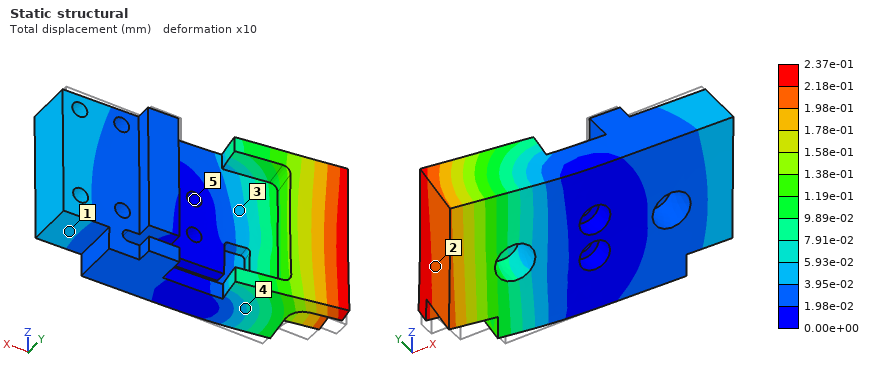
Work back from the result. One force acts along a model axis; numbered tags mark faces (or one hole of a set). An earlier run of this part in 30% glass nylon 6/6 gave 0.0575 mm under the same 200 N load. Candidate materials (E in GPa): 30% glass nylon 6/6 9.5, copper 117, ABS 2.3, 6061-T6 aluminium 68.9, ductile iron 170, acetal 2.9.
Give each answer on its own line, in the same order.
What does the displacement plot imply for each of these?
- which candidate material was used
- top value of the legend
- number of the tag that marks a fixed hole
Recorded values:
ABS
2.37e-01 mm
5
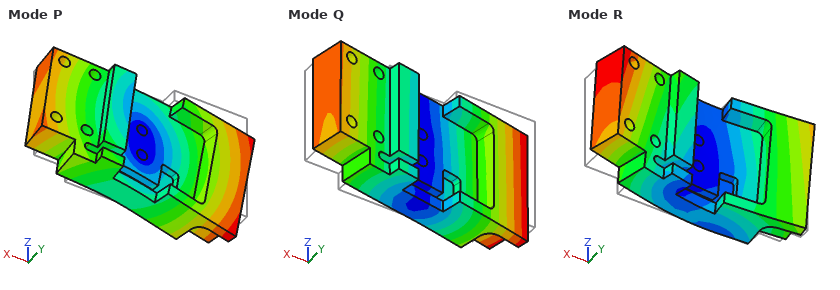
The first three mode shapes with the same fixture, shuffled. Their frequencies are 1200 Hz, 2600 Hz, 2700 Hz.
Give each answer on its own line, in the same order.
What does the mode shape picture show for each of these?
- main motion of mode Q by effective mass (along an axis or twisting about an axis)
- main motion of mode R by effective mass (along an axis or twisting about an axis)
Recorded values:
twisting about Z
along Y
